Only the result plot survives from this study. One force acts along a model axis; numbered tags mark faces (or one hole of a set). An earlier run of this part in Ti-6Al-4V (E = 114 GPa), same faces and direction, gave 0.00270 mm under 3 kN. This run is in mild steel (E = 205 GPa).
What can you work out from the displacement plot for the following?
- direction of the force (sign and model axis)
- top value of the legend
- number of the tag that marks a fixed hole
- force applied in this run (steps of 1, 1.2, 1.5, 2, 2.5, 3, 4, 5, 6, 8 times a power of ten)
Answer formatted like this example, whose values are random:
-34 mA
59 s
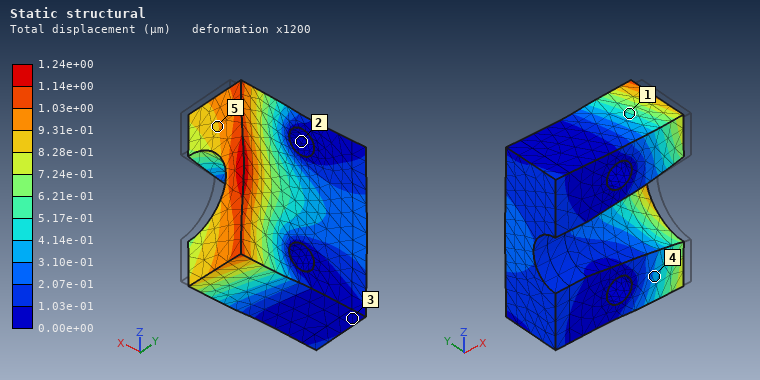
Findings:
-X
1.24e+00 µm
2
2.5 kN
